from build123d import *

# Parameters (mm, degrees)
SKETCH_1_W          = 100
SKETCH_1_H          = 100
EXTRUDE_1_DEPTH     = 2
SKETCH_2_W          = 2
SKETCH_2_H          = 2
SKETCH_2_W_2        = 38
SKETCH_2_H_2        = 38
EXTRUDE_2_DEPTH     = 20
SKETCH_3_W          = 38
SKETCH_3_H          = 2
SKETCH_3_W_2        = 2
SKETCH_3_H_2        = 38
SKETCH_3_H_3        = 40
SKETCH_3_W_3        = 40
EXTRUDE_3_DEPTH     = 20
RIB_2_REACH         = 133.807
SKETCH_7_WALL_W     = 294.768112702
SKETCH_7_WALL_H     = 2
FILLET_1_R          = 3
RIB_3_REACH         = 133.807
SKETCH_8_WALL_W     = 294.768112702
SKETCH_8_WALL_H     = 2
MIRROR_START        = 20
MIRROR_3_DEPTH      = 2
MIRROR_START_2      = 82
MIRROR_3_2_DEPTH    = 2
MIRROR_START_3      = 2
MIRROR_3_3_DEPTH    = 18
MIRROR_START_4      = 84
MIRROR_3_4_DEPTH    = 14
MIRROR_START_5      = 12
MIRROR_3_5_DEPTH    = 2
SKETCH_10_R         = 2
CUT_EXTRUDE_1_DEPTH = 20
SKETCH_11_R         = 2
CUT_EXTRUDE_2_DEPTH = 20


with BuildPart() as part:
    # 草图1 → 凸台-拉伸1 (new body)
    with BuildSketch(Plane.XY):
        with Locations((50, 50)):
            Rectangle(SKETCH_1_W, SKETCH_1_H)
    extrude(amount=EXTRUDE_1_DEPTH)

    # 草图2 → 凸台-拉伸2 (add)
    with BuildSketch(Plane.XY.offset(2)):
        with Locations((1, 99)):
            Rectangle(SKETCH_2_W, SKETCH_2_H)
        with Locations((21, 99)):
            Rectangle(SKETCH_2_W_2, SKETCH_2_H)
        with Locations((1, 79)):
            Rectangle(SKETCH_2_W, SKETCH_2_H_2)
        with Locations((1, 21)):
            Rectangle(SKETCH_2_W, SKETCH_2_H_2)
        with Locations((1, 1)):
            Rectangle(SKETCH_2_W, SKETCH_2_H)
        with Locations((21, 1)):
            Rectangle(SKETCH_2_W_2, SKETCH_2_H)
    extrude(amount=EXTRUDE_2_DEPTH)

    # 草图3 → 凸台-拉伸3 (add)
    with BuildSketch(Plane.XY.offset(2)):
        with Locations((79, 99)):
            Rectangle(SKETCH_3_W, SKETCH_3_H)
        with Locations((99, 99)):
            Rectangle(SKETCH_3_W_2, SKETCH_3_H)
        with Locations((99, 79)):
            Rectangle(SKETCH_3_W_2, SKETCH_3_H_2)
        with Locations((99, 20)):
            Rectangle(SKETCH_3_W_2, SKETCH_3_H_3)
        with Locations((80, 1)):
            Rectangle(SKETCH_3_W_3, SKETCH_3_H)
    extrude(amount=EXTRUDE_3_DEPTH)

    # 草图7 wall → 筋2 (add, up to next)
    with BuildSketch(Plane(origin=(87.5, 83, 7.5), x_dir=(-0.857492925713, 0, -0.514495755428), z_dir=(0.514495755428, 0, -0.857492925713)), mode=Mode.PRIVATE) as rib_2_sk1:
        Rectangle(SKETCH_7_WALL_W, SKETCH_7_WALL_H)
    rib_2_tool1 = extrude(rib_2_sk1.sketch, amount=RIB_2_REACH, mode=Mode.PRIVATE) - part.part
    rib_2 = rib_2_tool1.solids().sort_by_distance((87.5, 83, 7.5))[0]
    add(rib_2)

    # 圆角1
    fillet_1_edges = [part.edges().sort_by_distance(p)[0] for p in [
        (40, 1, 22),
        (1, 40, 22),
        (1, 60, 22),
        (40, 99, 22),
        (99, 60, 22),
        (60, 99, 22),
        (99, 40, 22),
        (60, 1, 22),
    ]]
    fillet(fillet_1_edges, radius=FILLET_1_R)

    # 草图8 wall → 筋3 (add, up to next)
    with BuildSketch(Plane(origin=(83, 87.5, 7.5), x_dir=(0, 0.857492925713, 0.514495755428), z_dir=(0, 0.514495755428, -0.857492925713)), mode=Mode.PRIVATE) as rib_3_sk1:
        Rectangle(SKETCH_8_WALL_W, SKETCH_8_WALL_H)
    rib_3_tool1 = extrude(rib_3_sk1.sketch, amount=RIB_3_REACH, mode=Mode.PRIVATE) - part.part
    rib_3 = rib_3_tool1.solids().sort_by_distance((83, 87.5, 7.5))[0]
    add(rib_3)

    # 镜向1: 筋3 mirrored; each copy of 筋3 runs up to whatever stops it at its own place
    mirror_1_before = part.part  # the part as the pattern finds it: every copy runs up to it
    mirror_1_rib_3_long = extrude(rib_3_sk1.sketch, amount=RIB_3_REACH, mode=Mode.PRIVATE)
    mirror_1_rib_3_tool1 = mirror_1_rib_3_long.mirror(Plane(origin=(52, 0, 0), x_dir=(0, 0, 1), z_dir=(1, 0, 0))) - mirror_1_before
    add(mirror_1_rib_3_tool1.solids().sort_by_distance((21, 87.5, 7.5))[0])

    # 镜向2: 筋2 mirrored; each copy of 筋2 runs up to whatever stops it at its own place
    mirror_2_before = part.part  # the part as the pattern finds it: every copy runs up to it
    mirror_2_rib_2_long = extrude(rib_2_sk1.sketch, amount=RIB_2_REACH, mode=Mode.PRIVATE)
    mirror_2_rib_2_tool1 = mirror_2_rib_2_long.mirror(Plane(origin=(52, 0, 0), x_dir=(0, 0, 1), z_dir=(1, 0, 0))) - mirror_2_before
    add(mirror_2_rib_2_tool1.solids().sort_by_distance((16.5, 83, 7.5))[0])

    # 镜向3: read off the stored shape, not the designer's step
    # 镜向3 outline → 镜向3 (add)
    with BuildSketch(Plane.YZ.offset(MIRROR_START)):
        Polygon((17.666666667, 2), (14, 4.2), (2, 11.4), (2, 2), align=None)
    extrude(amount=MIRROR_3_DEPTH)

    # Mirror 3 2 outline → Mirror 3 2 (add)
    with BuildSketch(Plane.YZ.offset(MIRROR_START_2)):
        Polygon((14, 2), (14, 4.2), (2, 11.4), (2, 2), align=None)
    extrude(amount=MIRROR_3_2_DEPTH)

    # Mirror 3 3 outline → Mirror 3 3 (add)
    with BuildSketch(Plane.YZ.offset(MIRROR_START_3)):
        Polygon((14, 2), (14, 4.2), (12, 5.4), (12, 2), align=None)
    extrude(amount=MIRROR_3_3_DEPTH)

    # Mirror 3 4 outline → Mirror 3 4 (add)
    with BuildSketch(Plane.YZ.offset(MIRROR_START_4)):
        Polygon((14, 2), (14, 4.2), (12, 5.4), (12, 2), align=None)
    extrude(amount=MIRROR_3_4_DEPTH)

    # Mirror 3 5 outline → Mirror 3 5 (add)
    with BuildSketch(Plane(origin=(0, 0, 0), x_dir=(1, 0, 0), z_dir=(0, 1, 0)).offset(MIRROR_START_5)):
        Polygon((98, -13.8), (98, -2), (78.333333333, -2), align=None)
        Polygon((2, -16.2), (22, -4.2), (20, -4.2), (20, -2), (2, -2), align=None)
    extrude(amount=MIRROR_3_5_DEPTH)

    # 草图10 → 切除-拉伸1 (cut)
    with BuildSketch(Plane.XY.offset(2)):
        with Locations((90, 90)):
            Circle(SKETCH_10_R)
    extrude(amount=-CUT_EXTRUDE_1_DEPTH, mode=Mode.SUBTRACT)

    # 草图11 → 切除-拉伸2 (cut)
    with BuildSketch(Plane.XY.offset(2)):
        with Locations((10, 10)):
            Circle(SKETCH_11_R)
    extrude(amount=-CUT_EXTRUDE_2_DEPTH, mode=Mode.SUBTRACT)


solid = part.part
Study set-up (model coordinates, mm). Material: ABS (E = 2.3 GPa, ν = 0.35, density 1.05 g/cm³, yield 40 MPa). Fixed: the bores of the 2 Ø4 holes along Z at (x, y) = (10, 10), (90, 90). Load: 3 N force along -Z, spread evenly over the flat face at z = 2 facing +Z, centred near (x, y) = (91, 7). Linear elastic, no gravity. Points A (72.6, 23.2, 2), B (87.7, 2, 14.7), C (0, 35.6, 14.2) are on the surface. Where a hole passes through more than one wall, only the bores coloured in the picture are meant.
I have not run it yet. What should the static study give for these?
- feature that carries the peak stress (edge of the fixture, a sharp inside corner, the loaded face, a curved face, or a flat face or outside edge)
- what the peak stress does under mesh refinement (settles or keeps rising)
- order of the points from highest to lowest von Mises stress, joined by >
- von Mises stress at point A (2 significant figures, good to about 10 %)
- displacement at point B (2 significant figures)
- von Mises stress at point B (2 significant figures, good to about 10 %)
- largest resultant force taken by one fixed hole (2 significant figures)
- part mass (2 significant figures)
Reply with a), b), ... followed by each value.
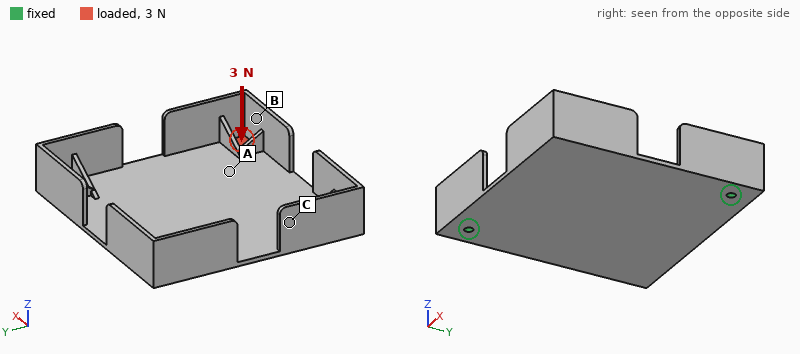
a) edge of the fixture
b) keeps rising
c) A > B > C
d) 1.3 MPa
e) 1.3 mm
f) 0.48 MPa
g) 2.0 N
h) 36 g
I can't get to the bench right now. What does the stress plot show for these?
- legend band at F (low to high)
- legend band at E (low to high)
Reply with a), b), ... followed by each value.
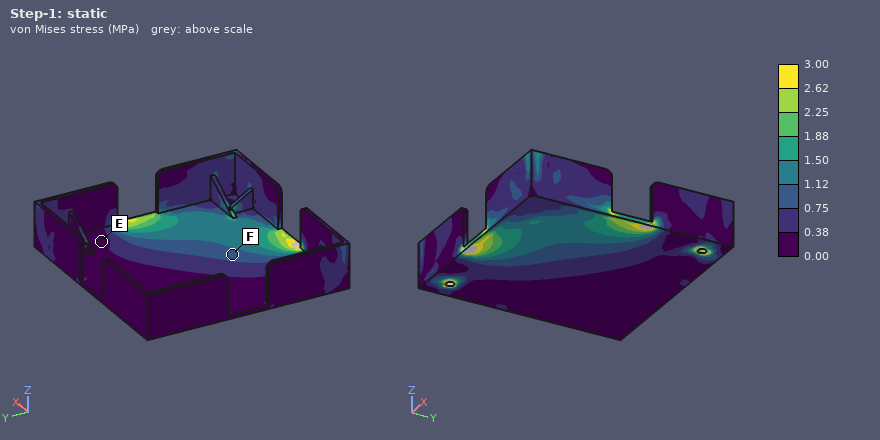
a) 0.75 to 1.12 MPa
b) 0.00 to 0.38 MPa
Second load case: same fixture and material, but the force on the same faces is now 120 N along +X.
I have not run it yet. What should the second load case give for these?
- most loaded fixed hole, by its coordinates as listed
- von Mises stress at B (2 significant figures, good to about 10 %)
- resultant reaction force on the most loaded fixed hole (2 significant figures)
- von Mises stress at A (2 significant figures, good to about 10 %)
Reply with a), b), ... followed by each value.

a) (10, 10)
b) 0.56 MPa
c) 100 N
d) 2.6 MPa
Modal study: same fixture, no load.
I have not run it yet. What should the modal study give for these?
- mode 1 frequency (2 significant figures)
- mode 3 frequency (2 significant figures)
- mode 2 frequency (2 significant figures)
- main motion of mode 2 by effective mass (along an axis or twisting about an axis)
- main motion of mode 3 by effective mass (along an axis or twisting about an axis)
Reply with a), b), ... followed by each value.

a) 110 Hz
b) 300 Hz
c) 120 Hz
d) along Z
e) along Z
